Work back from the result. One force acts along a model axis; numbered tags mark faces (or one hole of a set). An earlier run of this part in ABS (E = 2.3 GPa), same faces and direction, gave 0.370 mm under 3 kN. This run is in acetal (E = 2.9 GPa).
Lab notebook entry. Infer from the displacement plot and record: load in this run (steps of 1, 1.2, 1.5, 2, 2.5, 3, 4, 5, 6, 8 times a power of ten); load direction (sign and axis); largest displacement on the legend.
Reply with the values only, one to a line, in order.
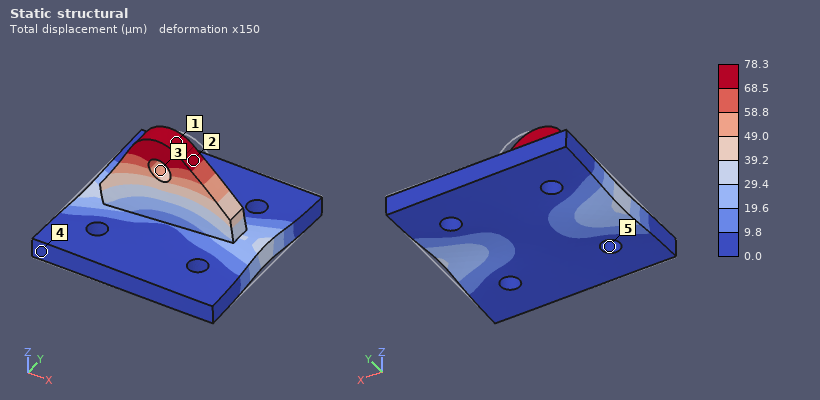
800 N
-X
78.3 µm
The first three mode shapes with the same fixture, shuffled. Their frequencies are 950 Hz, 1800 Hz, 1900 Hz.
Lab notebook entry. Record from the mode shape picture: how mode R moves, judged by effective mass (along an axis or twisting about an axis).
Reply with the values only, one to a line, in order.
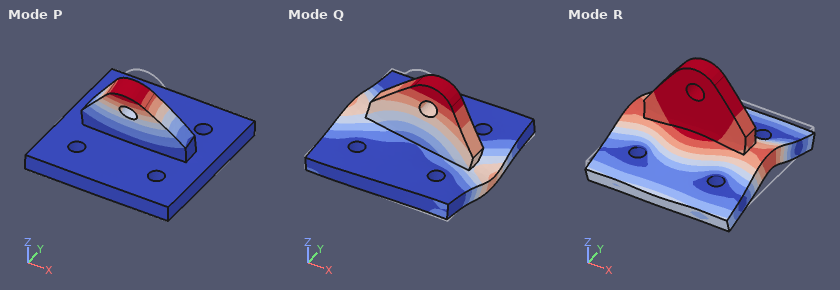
along Z
